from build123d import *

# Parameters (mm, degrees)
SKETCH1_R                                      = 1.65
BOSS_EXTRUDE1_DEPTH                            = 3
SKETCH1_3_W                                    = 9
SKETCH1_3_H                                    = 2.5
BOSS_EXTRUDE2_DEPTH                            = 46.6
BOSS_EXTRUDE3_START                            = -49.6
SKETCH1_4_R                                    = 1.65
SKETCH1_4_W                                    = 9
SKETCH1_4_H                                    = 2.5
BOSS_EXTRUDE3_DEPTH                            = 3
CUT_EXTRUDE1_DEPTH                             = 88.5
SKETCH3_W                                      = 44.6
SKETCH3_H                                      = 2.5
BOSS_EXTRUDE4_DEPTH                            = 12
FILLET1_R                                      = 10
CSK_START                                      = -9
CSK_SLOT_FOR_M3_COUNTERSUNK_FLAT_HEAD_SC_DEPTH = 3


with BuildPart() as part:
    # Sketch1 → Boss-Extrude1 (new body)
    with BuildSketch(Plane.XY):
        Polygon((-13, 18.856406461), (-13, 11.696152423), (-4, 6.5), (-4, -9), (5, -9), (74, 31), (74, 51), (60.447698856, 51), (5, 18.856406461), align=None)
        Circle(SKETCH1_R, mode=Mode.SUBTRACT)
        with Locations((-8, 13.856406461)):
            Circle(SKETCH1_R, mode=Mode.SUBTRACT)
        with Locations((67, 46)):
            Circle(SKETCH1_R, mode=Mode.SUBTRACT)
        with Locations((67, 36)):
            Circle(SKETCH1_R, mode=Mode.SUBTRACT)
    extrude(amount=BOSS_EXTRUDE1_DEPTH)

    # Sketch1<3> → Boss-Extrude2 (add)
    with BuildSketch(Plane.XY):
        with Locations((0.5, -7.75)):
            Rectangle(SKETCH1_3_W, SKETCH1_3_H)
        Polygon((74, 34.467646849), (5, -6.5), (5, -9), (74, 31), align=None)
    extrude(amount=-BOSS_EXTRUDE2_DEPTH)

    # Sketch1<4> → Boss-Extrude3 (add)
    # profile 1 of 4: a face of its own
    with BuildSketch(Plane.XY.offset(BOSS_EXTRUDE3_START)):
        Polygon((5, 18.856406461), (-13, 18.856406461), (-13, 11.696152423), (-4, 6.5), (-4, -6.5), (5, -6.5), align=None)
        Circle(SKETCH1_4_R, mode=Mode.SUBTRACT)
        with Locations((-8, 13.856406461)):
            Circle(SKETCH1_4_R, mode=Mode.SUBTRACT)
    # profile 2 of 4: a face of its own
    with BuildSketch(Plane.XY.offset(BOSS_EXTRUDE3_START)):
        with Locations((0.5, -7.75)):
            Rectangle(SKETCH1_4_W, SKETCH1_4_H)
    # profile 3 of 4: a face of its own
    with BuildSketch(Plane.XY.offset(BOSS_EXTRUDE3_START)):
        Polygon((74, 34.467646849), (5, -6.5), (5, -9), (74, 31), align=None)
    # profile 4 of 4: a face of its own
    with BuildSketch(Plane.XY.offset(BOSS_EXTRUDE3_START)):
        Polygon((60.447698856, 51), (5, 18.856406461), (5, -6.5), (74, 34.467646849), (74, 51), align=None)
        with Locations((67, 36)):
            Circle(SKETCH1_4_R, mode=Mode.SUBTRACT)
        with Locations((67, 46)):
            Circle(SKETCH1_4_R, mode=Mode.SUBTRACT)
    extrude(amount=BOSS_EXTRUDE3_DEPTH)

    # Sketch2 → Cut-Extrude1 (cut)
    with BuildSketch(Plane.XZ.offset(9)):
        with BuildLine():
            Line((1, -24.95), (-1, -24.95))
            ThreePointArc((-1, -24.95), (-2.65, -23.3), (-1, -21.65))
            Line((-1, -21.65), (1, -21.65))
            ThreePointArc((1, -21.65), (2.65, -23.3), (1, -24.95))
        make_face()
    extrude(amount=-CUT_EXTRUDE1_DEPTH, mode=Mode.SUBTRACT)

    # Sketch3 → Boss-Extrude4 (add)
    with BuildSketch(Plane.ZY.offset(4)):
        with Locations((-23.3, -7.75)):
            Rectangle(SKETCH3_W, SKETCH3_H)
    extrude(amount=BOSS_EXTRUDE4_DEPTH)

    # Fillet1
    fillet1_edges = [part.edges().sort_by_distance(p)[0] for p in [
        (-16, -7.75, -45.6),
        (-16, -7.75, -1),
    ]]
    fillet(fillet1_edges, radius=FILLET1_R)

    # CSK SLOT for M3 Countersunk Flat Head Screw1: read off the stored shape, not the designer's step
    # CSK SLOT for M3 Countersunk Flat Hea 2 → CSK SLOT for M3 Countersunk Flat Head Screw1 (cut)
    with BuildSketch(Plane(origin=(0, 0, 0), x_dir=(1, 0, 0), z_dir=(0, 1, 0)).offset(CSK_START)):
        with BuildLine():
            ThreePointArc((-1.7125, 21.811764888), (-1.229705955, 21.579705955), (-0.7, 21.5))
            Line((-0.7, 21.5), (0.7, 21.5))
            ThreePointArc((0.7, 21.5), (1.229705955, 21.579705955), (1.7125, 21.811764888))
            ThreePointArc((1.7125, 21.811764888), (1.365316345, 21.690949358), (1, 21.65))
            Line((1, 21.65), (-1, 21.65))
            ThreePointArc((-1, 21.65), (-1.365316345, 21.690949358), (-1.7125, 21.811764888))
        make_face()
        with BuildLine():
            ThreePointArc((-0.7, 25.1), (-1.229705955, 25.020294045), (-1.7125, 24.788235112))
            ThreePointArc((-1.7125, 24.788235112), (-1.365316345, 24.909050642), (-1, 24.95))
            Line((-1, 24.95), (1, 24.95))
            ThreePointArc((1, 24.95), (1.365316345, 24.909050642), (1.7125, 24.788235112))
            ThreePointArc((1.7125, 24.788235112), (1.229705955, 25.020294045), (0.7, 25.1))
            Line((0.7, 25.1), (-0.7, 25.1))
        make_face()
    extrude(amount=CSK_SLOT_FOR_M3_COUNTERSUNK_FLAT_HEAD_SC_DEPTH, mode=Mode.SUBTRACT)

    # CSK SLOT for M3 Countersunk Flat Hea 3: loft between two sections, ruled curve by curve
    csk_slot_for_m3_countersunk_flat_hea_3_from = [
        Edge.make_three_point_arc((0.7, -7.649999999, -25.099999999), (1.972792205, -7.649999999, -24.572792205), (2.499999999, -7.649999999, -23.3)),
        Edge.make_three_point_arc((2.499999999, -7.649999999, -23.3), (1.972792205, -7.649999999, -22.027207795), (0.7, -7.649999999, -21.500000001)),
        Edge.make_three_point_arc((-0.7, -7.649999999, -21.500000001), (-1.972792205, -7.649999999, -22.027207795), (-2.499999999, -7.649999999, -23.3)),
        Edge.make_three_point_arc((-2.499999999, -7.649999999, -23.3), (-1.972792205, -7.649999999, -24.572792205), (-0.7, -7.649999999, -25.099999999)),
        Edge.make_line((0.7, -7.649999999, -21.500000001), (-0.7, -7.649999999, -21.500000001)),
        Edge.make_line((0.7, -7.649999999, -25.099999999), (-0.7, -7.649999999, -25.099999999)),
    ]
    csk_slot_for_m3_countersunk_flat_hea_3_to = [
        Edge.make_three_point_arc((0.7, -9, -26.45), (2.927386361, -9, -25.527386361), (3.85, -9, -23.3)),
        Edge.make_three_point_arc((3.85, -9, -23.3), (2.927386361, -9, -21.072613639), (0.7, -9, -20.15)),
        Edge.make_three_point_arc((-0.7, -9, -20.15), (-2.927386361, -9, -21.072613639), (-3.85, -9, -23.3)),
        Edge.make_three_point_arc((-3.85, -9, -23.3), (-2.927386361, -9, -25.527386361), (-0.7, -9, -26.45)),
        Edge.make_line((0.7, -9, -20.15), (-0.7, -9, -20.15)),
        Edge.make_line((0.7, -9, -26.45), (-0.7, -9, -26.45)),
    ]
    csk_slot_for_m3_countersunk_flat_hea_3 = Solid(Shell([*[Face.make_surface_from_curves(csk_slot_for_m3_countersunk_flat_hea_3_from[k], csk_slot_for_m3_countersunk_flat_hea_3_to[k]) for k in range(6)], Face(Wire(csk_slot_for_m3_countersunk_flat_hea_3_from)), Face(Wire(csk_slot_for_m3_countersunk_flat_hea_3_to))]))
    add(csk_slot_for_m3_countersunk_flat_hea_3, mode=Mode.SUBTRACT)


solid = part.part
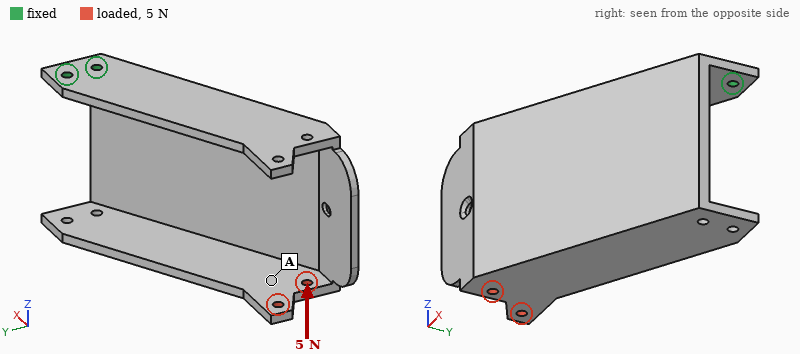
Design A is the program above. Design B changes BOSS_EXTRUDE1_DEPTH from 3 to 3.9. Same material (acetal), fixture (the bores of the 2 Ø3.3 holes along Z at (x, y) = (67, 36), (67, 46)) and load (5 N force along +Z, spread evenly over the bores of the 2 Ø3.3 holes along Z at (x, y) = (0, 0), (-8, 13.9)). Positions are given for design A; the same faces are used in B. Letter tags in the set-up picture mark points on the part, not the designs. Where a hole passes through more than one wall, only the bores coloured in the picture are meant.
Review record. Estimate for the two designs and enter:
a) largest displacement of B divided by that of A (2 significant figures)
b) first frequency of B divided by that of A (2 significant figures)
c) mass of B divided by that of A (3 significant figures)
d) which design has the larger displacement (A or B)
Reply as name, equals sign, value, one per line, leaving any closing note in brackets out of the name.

largest displacement of B divided by that of A = 0.68
first frequency of B divided by that of A = 1.2
mass of B divided by that of A = 1.08
which design has the larger displacement = A
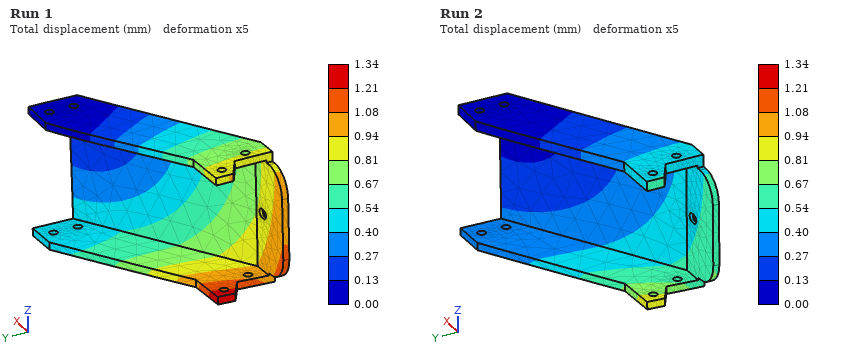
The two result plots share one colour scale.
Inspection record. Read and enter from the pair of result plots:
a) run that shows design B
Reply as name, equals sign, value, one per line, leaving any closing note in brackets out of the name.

run that shows design B = Run 2
